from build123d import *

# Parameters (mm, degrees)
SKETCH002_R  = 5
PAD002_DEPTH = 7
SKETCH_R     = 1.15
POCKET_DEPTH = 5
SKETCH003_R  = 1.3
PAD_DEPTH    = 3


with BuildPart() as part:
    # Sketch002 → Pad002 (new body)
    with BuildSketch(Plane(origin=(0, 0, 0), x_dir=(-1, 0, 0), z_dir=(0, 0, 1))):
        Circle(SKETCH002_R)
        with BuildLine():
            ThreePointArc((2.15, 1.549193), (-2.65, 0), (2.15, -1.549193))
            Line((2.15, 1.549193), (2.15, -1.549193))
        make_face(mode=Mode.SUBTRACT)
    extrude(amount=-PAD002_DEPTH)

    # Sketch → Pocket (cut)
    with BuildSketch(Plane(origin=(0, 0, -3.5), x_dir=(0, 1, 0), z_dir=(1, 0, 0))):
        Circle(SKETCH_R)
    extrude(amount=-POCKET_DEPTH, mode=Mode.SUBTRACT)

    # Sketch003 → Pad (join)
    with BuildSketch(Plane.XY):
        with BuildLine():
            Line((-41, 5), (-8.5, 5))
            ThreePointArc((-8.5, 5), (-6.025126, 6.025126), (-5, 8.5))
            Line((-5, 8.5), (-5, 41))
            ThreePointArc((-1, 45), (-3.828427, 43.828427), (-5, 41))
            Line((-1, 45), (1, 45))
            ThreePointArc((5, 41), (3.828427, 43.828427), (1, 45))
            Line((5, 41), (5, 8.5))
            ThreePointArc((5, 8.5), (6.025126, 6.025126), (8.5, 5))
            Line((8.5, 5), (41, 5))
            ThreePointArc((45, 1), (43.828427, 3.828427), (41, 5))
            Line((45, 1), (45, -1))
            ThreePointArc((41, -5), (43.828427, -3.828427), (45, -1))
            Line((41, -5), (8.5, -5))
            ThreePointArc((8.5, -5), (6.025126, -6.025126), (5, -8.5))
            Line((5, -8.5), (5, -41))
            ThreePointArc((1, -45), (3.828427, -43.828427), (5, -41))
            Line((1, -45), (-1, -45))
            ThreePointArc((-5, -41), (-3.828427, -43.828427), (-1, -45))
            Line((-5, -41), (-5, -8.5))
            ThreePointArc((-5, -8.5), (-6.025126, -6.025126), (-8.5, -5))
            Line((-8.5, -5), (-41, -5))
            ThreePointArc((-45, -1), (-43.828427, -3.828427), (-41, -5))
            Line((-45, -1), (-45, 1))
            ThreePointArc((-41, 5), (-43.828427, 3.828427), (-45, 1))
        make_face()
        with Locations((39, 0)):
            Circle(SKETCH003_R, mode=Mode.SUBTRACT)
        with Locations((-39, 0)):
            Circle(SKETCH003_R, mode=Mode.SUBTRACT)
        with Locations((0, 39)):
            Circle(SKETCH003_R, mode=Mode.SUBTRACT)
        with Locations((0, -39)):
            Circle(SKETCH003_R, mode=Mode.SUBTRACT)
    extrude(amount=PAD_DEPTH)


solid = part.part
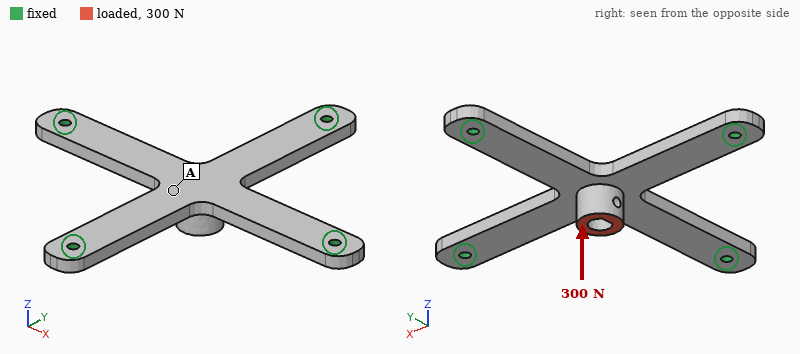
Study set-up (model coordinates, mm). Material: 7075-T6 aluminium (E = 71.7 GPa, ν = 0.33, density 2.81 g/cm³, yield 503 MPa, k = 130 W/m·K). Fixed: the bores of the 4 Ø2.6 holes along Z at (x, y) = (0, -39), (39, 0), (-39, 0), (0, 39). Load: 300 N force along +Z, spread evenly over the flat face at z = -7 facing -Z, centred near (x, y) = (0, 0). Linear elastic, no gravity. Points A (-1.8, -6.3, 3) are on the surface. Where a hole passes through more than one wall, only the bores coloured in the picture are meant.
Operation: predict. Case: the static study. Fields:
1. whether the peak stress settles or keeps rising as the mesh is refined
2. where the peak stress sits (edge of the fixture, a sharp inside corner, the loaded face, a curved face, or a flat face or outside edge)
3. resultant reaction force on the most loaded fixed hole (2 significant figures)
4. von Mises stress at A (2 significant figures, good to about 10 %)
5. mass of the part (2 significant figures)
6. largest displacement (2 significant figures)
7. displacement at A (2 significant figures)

keeps rising
edge of the fixture
76 N
56 MPa
15 g
0.16 mm
0.16 mm
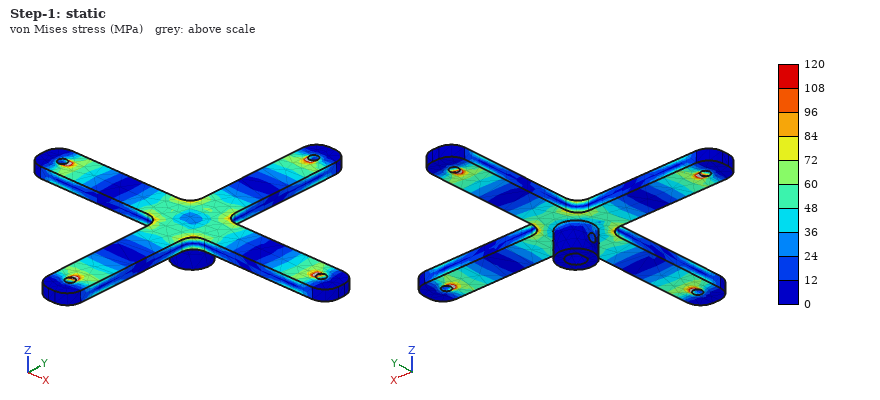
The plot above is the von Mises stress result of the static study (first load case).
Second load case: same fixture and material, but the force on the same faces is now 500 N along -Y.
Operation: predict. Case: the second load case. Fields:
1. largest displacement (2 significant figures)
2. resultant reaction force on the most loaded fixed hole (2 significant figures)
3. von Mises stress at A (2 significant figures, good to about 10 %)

77 µm
250 N
61 MPa
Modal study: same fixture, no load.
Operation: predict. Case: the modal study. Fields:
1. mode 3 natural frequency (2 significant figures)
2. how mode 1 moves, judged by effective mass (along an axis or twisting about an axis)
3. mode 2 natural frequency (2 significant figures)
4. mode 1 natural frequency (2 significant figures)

7100 Hz
along Z
7100 Hz
2800 Hz
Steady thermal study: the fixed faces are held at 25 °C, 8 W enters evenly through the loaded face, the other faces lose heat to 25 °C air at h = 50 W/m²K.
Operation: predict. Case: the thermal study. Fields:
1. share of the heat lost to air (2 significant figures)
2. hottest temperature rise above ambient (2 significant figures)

21 %
24 K
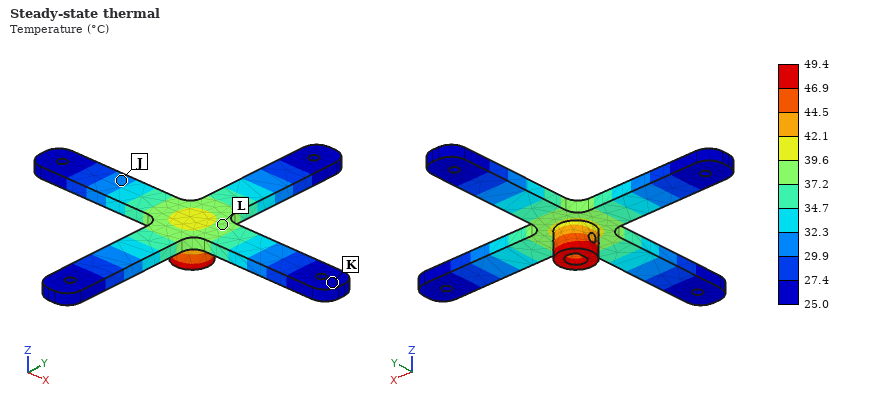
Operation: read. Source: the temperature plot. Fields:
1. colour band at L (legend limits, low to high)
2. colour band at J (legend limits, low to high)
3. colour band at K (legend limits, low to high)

37.2 to 39.6 °C
29.9 to 32.3 °C
25.0 to 27.4 °C
